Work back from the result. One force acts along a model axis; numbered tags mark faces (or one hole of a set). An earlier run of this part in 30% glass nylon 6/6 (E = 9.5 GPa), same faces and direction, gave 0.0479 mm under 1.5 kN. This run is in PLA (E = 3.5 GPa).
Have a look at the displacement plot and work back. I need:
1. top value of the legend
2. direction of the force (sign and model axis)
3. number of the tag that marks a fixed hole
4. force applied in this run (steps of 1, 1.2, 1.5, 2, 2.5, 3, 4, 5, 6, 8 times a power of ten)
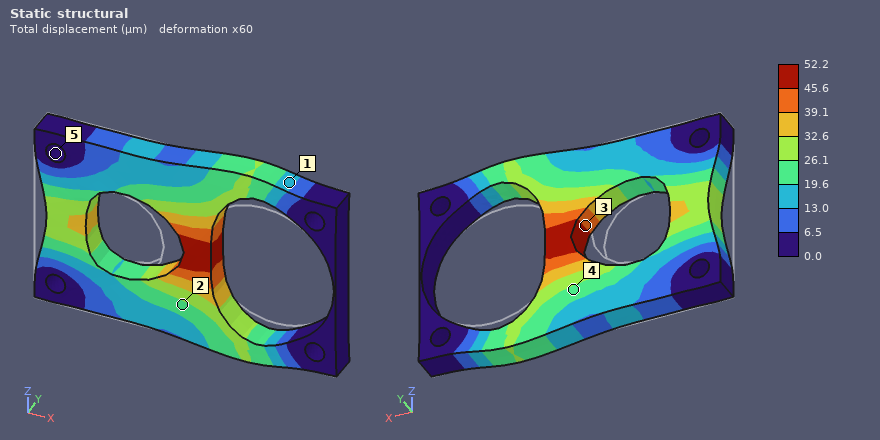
52.2 µm
+X
5
600 N
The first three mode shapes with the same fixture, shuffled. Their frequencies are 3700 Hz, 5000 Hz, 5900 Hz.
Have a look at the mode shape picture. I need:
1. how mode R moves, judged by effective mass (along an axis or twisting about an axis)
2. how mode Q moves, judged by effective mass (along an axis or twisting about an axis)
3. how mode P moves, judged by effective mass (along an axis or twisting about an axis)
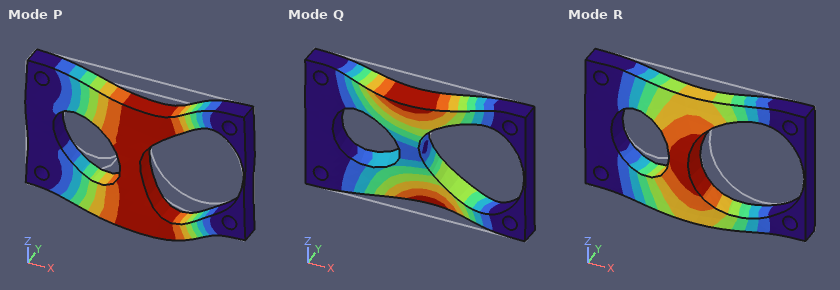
along Y
twisting about X
along Z
